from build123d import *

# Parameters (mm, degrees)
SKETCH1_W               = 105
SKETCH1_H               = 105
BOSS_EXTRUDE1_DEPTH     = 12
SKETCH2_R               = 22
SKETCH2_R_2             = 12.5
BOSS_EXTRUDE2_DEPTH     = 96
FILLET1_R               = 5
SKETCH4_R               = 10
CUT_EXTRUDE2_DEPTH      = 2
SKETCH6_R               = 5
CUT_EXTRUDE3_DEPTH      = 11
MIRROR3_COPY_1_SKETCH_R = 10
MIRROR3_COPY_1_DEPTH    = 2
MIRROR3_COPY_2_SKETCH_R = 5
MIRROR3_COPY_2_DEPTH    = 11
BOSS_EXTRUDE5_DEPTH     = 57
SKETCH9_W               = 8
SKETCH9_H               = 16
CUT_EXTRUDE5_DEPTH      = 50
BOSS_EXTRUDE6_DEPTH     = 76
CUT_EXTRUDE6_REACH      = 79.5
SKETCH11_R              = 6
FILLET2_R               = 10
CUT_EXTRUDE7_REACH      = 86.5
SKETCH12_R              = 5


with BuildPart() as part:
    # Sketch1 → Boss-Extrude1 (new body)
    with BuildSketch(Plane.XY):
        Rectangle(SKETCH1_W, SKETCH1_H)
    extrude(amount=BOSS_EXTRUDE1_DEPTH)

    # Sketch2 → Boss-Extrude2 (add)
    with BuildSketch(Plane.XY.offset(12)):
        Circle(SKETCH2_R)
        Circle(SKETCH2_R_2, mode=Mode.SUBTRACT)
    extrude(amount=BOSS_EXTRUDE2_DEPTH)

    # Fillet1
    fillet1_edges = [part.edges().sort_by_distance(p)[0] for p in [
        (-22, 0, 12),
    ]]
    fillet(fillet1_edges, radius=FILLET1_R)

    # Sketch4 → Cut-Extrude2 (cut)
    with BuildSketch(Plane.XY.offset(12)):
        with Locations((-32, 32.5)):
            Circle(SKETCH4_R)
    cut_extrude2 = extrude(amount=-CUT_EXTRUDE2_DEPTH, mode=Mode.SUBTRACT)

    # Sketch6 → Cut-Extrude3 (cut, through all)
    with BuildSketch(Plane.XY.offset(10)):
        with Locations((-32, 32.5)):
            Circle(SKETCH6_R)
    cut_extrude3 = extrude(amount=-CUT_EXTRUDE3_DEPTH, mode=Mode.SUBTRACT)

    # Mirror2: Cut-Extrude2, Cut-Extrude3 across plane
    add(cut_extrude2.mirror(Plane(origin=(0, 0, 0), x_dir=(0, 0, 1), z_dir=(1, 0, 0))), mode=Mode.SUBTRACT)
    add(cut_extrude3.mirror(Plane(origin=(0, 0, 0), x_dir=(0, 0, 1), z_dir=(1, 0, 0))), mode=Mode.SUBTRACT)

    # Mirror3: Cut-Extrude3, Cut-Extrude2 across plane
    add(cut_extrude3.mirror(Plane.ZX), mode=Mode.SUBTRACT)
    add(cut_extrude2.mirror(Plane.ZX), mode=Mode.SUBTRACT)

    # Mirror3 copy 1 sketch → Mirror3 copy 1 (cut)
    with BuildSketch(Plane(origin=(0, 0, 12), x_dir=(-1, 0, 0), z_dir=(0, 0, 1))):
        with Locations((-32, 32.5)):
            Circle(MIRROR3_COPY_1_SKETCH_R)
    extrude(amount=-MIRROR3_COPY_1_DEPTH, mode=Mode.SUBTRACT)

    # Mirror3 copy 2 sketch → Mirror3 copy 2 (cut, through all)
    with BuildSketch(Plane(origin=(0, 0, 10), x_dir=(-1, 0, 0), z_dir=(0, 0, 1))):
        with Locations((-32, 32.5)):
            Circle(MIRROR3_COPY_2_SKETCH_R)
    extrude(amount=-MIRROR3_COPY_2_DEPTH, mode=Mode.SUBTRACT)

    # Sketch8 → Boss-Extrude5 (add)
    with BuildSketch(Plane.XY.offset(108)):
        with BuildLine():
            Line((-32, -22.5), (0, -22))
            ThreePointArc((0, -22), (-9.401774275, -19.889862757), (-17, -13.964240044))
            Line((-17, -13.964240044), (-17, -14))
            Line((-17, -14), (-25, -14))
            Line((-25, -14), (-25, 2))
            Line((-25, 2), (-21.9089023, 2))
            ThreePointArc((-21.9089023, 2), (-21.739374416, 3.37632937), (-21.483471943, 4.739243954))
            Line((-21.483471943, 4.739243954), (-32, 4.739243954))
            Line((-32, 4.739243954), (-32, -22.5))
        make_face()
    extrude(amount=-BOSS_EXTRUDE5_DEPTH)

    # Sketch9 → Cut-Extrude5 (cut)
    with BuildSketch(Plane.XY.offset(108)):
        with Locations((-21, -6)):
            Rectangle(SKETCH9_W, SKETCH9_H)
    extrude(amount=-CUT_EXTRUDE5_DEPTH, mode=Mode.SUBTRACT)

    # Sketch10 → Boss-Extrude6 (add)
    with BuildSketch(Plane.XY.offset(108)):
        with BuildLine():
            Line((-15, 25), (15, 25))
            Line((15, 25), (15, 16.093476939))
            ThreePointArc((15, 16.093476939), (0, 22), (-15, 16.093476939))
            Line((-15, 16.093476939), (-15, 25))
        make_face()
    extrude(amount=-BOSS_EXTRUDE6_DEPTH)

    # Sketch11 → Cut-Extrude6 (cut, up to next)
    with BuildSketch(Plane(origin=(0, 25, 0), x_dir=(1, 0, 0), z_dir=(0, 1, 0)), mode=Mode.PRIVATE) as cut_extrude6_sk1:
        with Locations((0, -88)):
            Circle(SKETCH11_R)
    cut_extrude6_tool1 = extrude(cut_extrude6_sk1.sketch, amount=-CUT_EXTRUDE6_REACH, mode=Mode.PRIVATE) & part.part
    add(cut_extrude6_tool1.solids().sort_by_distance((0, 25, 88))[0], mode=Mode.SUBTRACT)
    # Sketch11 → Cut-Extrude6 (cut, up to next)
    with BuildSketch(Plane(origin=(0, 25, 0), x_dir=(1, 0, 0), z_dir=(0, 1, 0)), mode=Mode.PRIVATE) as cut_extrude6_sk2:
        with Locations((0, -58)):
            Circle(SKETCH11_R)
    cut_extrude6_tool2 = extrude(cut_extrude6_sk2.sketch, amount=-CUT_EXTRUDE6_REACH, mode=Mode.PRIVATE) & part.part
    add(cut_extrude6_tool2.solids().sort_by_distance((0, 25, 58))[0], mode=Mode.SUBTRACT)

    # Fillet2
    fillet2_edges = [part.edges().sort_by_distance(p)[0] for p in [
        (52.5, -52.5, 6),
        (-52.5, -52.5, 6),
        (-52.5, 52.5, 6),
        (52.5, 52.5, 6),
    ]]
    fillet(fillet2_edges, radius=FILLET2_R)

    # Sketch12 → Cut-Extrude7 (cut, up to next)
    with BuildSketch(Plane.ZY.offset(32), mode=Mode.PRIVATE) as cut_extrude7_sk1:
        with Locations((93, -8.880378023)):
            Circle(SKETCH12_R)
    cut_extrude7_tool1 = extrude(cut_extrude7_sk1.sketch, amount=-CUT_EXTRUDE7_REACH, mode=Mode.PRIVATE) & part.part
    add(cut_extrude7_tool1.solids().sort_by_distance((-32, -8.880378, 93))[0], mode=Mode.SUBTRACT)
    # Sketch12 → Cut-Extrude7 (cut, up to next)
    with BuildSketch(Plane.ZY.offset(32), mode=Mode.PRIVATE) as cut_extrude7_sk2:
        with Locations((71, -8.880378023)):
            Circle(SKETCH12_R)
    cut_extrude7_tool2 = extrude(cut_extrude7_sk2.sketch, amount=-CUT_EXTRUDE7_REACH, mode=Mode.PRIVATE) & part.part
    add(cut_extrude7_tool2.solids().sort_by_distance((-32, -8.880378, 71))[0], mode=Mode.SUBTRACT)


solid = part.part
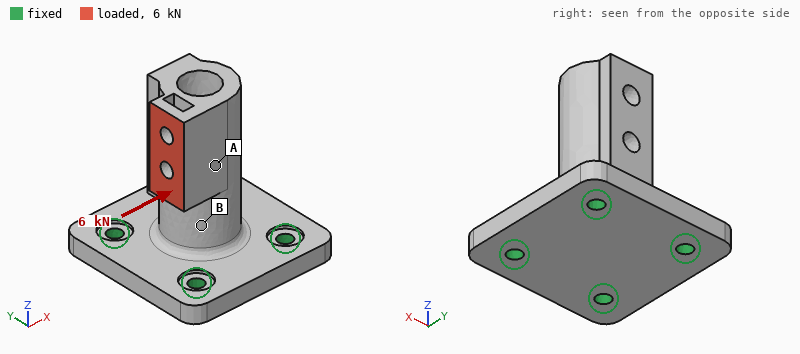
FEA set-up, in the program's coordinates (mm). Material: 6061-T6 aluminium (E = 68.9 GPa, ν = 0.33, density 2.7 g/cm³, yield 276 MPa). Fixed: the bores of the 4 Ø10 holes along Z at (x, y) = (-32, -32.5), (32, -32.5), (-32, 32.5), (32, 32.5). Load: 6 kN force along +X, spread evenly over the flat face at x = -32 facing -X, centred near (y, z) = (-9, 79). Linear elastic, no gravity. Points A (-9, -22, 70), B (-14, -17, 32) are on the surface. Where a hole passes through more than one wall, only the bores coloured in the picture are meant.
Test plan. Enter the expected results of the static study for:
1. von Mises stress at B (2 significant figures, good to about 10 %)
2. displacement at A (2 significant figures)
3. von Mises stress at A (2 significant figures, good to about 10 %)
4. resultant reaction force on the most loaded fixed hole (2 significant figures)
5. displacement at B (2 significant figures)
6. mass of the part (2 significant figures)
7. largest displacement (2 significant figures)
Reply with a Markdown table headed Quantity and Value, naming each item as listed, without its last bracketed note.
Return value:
| Quantity | Value |
|---|---|
| von Mises stress at B | 29 MPa |
| displacement at A | 0.14 mm |
| von Mises stress at A | 14 MPa |
| resultant reaction force on the most loaded fixed hole | 4.3 kN |
| displacement at B | 0.049 mm |
| mass of the part | 670 g |
| largest displacement | 0.25 mm |
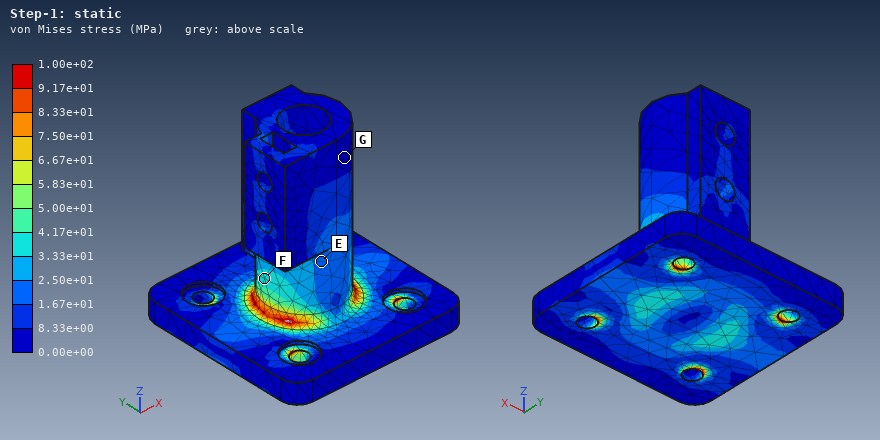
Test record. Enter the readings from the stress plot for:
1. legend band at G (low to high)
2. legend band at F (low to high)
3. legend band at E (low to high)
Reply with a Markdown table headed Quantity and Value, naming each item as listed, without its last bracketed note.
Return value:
| Quantity | Value |
|---|---|
| legend band at G | 0.00e+00 to 8.33e+00 MPa |
| legend band at F | 3.33e+01 to 4.17e+01 MPa |
| legend band at E | 1.67e+01 to 2.50e+01 MPa |
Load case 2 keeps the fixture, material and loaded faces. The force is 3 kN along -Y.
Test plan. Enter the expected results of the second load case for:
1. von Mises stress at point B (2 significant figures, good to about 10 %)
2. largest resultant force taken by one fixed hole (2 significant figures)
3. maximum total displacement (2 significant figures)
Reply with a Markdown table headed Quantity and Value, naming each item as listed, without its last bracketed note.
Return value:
| Quantity | Value |
|---|---|
| von Mises stress at point B | 21 MPa |
| largest resultant force taken by one fixed hole | 2.2 kN |
| maximum total displacement | 0.15 mm |
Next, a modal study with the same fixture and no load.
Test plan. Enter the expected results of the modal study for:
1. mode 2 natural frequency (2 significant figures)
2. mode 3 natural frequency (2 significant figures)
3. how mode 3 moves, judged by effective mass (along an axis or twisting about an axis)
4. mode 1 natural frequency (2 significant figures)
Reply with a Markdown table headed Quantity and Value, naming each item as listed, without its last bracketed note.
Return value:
| Quantity | Value |
|---|---|
| mode 2 natural frequency | 2000 Hz |
| mode 3 natural frequency | 5200 Hz |
| how mode 3 moves, judged by effective mass | along Z |
| mode 1 natural frequency | 1900 Hz |
